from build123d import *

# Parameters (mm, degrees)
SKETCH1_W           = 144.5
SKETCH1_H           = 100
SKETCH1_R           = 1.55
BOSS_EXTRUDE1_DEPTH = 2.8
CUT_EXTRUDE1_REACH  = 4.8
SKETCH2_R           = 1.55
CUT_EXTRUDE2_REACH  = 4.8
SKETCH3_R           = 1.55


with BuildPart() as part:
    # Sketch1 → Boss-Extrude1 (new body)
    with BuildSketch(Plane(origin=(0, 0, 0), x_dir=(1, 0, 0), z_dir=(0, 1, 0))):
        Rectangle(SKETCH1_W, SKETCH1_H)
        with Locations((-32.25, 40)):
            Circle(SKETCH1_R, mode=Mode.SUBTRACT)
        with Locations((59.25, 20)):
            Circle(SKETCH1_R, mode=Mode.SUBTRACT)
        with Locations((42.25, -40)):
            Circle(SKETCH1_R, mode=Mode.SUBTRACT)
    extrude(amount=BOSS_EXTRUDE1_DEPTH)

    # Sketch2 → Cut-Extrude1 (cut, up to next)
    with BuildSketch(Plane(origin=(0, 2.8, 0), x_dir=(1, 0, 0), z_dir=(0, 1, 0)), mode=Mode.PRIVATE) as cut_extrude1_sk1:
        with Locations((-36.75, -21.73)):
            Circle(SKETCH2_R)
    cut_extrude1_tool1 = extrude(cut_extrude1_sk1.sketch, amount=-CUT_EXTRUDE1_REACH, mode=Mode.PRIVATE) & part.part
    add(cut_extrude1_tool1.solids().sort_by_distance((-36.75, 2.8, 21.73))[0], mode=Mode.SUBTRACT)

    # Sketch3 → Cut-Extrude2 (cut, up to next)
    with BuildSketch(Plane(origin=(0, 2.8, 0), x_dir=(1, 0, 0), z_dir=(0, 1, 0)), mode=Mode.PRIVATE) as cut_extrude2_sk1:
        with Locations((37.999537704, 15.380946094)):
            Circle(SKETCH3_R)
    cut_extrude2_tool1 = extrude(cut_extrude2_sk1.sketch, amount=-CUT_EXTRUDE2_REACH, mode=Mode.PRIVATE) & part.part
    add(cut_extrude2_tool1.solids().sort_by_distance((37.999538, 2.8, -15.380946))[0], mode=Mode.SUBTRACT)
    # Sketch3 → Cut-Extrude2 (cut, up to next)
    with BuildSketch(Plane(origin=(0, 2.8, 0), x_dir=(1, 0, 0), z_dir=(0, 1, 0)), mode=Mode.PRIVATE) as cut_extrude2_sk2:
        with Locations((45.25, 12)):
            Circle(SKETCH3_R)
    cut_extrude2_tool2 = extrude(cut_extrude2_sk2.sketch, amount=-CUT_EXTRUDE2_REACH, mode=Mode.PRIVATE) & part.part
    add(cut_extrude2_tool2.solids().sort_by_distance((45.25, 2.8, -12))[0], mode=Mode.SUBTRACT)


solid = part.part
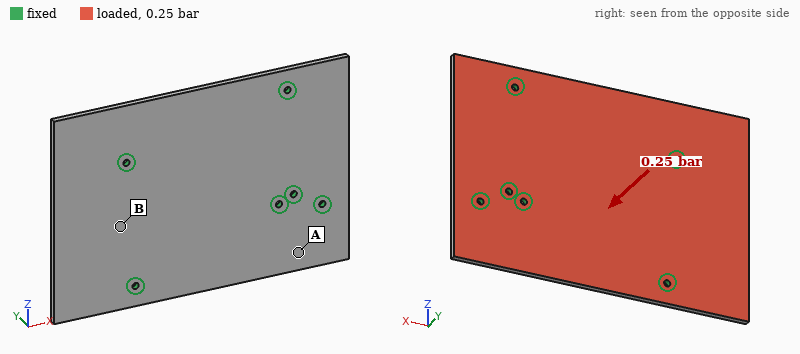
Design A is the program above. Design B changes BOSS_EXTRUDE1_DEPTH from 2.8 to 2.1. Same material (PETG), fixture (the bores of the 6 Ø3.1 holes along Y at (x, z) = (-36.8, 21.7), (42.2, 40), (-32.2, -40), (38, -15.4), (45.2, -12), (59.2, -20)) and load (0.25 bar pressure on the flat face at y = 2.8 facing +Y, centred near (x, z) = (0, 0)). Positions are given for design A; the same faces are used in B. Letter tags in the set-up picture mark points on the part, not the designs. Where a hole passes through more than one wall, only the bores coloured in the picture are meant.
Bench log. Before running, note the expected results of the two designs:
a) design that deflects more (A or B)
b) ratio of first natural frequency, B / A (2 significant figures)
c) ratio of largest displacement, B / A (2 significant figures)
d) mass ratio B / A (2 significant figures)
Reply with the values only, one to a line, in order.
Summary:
B
0.77
2.3
0.75
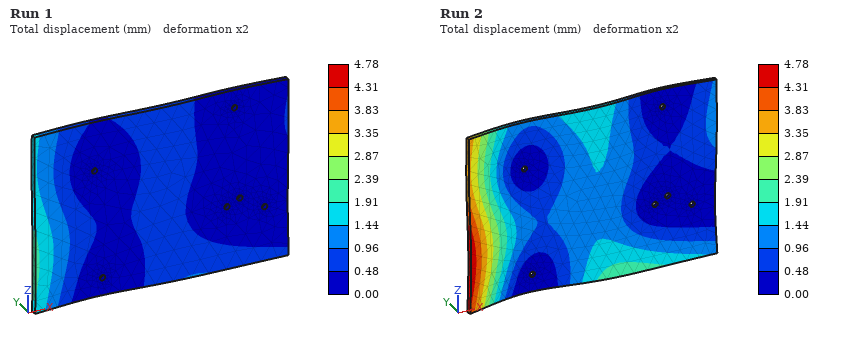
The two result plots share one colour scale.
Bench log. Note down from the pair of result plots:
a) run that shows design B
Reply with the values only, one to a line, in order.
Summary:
Run 2
